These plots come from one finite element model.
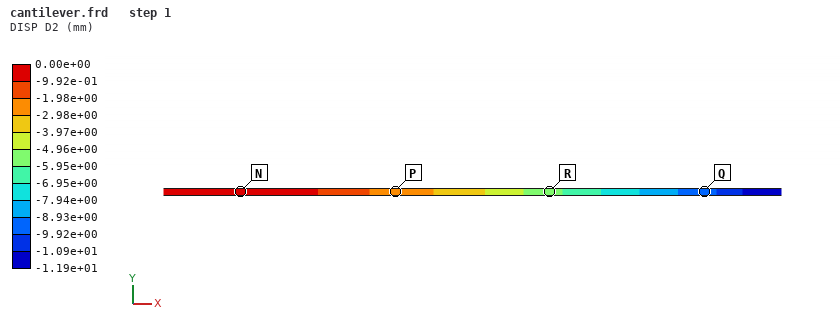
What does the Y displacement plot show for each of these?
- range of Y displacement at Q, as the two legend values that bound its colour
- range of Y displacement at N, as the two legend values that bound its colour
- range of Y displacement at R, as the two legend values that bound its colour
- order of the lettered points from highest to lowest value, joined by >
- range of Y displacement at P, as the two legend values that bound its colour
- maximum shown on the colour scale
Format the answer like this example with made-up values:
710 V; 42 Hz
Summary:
-9.92e+00 to -8.93e+00 mm; -9.92e-01 to 0.00e+00 mm; -5.95e+00 to -4.96e+00 mm; N > P > R > Q; -2.98e+00 to -1.98e+00 mm; 0.00e+00 mm
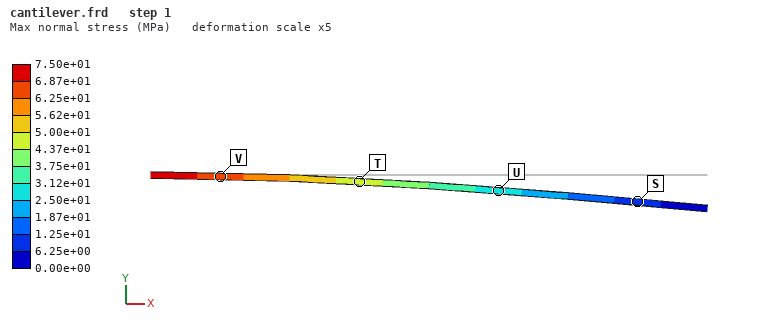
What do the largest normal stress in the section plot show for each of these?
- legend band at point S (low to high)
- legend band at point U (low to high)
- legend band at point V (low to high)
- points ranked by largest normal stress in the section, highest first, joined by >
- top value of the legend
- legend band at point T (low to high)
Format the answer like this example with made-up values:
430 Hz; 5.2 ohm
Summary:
6.25e+00 to 1.25e+01 MPa; 2.50e+01 to 3.12e+01 MPa; 6.25e+01 to 6.87e+01 MPa; V > T > U > S; 7.50e+01 MPa; 4.37e+01 to 5.00e+01 MPa
